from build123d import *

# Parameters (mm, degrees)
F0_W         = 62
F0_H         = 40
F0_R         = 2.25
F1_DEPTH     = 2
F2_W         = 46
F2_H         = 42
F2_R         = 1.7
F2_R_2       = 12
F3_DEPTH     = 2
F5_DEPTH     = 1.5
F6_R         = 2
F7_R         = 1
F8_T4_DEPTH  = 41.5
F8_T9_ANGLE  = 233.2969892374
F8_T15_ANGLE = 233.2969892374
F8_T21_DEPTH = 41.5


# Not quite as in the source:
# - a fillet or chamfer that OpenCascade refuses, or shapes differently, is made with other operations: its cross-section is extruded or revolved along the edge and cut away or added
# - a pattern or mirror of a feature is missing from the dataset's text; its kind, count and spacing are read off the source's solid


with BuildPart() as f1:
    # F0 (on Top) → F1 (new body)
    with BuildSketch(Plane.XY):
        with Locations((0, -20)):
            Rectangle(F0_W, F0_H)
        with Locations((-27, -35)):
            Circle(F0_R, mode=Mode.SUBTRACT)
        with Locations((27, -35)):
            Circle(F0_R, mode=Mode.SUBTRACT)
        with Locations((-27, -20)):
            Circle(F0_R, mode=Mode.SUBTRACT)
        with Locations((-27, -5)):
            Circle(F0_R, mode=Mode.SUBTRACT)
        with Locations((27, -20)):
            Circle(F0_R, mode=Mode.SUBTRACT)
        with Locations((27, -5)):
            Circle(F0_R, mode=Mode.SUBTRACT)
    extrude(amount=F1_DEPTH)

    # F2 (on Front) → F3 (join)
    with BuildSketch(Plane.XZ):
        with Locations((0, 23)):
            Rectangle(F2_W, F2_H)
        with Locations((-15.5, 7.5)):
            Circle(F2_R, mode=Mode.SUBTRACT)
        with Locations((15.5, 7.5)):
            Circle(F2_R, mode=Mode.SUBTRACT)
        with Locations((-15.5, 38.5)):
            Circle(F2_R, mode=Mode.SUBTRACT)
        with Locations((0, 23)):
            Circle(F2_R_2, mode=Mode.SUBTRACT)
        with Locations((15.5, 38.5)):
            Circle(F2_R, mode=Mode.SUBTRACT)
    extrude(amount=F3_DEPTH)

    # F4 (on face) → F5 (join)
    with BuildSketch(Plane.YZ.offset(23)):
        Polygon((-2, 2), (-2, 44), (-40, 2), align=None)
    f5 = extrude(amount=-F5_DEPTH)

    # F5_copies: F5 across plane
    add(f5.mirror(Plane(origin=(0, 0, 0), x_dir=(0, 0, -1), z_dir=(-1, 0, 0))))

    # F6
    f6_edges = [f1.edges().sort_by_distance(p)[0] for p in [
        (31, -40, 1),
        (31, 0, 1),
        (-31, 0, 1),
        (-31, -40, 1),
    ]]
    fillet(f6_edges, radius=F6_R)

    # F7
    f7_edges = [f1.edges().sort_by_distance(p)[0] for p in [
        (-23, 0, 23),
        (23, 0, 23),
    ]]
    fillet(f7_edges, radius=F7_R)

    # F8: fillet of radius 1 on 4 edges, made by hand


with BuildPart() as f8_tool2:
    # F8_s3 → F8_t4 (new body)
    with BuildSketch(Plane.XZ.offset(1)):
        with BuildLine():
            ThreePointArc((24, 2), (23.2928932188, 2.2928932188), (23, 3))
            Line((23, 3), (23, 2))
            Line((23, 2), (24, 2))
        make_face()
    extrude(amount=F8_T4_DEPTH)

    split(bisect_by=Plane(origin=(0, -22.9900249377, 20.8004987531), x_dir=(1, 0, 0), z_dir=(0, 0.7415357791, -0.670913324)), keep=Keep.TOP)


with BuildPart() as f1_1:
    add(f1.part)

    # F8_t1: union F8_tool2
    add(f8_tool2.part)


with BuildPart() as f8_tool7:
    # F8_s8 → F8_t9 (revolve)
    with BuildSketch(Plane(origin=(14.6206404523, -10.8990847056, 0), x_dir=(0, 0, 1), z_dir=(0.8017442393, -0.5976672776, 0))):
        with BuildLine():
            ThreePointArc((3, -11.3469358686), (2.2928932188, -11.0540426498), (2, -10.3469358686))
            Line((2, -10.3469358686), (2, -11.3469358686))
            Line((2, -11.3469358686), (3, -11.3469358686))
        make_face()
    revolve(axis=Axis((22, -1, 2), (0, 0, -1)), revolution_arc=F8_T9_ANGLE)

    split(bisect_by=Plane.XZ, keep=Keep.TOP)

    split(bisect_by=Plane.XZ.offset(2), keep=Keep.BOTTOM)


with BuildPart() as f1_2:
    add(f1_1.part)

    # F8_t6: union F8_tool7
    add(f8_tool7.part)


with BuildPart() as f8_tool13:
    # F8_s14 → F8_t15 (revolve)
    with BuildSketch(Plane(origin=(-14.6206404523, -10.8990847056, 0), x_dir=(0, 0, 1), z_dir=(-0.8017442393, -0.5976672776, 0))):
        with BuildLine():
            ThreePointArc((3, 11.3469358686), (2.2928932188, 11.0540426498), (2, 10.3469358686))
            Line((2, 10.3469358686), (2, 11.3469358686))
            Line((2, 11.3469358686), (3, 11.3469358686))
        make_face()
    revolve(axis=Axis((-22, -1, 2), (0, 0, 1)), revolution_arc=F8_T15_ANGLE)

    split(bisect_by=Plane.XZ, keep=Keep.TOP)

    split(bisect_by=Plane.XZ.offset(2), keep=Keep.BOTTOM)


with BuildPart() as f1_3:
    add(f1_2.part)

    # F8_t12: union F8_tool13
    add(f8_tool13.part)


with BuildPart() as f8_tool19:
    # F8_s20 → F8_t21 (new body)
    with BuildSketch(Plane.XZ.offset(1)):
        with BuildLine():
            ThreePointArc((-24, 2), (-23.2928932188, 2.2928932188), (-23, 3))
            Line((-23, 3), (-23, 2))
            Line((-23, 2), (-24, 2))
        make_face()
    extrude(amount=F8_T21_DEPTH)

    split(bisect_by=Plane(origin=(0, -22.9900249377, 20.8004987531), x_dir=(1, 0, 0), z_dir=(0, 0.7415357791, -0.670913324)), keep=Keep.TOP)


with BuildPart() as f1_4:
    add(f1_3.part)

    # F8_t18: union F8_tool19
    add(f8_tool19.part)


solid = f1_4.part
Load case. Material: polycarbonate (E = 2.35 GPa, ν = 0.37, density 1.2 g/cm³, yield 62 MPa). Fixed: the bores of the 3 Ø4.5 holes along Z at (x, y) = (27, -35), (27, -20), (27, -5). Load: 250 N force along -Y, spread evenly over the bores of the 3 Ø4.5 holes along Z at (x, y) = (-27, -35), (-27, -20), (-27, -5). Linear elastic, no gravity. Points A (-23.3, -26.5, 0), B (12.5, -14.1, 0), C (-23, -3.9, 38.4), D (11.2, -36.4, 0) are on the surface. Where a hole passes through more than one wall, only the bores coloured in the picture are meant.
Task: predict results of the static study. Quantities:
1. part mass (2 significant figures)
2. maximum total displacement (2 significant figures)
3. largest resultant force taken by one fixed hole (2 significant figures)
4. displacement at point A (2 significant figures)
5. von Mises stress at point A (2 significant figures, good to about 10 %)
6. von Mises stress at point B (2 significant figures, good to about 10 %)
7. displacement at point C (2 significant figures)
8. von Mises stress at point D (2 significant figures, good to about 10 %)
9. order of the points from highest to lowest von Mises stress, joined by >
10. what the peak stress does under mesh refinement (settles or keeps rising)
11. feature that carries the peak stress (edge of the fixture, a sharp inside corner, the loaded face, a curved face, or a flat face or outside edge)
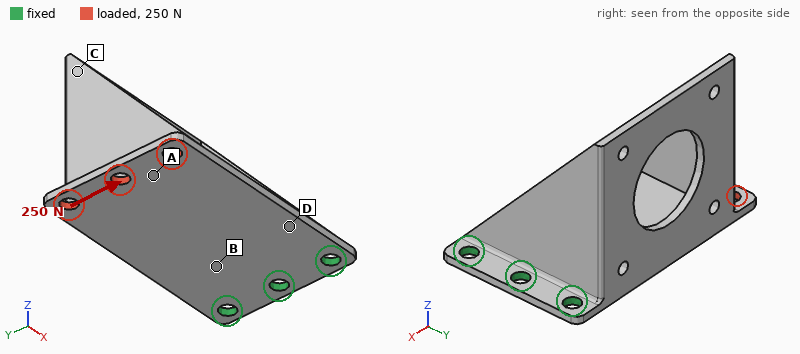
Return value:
12 g
0.94 mm
430 N
0.73 mm
5.4 MPa
8.9 MPa
0.68 mm
13 MPa
D > B > A > C
keeps rising
edge of the fixture
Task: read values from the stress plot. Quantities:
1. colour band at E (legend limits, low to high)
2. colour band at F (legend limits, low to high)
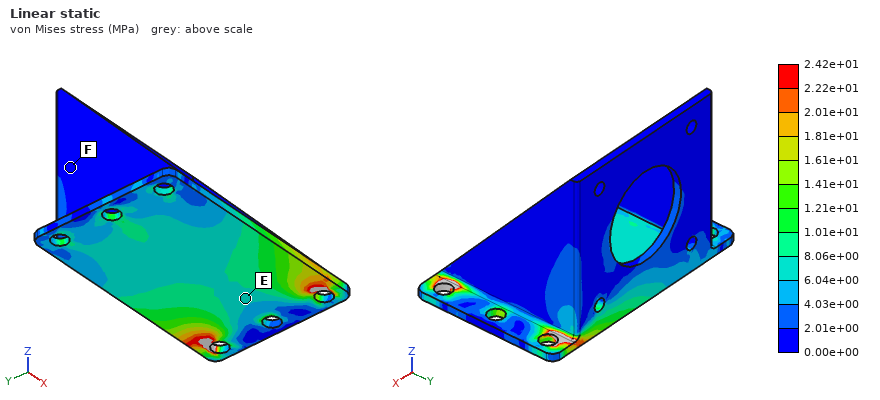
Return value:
6.04e+00 to 8.06e+00 MPa
0.00e+00 to 2.01e+00 MPa
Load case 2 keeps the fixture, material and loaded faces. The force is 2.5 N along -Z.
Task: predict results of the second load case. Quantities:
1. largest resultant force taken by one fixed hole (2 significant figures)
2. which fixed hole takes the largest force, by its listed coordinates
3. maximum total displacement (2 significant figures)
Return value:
2.7 N
(27, -20)
0.89 mm
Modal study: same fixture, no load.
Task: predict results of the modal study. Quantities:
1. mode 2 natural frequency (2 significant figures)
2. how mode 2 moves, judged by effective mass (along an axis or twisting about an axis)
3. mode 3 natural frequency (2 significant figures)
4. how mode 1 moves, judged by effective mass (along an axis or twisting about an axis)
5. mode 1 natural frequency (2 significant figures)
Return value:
260 Hz
along Y
890 Hz
along Z
130 Hz
